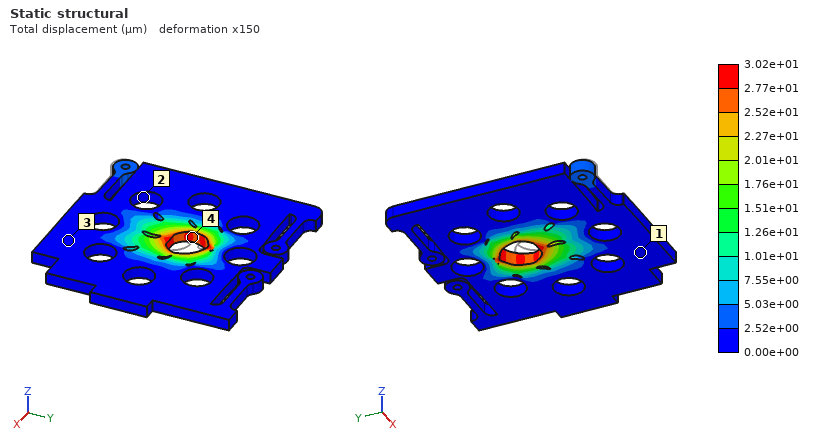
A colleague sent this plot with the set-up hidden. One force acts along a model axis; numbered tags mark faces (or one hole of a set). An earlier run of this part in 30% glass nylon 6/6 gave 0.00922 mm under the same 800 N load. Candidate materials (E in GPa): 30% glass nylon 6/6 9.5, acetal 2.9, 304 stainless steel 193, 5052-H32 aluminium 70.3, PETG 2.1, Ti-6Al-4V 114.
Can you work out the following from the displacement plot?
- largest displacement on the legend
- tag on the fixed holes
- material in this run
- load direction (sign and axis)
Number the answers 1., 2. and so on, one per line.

1. 3.02e+01 µm
2. 2
3. acetal
4. +Y
